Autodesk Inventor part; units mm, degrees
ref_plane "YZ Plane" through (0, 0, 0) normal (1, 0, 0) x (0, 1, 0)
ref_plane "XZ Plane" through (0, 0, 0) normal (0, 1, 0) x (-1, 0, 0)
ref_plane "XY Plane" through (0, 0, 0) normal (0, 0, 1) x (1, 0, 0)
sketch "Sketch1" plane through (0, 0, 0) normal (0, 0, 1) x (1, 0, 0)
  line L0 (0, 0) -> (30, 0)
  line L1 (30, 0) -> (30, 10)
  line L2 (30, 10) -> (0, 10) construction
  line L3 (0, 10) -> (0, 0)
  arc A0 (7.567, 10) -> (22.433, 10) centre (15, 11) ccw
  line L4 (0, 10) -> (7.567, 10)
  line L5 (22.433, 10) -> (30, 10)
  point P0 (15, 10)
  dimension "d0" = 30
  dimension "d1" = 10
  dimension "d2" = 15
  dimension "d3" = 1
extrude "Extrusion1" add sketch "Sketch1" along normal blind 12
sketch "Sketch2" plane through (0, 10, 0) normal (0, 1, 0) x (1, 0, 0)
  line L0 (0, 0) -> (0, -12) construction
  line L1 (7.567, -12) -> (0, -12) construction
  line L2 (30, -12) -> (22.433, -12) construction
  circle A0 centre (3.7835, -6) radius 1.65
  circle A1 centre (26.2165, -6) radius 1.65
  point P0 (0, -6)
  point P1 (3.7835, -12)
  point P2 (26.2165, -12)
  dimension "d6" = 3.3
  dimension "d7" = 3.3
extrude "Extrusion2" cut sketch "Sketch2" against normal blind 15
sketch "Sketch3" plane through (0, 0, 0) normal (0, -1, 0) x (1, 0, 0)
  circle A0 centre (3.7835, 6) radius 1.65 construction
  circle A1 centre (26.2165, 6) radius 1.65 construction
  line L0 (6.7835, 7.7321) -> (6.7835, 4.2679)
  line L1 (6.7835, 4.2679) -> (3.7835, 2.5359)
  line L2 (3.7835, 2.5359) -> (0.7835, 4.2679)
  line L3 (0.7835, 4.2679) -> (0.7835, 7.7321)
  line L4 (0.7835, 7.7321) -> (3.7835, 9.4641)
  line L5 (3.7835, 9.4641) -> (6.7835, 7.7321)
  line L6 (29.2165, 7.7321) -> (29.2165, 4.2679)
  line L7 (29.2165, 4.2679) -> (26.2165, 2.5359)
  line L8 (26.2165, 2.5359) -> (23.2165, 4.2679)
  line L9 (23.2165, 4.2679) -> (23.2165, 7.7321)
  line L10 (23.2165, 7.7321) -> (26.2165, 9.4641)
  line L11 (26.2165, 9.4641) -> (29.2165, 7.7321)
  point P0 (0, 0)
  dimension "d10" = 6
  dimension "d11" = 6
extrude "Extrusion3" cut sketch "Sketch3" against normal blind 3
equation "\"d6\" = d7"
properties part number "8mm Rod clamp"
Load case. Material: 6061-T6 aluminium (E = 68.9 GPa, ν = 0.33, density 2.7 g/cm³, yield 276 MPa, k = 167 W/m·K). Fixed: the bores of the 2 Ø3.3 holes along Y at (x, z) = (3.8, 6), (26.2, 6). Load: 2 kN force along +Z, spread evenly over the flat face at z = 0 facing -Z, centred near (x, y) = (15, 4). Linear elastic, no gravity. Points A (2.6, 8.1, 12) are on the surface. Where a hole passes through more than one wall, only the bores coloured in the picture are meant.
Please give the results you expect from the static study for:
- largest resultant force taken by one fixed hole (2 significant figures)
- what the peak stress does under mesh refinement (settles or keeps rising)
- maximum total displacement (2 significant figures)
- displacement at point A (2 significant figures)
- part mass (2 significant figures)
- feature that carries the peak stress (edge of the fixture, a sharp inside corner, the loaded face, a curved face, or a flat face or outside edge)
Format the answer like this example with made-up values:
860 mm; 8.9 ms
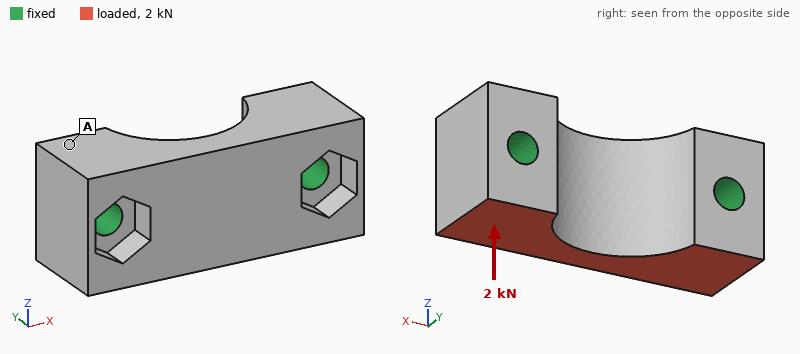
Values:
1.0 kN; keeps rising; 6.6 µm; 1.3 µm; 6.5 g; edge of the fixture
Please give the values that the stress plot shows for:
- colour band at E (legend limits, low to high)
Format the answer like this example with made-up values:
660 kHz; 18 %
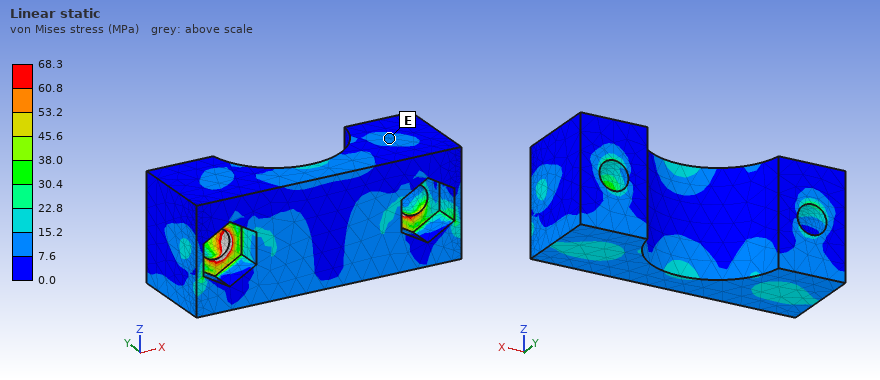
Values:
7.6 to 15.2 MPa
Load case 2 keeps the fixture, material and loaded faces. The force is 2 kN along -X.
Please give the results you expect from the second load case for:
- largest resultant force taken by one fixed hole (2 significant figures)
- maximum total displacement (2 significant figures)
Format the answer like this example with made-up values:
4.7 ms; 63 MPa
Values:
1.1 kN; 6.6 µm
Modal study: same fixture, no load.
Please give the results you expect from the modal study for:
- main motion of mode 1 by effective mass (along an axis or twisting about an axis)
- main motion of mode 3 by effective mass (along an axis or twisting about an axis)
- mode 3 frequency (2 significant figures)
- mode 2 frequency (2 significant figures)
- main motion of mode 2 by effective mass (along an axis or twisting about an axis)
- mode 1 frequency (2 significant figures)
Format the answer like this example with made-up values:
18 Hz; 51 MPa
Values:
along Z; twisting about X; 67 kHz; 56 kHz; along Y; 41 kHz
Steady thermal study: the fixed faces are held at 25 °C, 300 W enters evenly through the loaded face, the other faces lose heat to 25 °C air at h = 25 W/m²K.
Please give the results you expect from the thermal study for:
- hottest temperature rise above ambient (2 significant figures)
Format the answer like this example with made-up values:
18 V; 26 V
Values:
82 K
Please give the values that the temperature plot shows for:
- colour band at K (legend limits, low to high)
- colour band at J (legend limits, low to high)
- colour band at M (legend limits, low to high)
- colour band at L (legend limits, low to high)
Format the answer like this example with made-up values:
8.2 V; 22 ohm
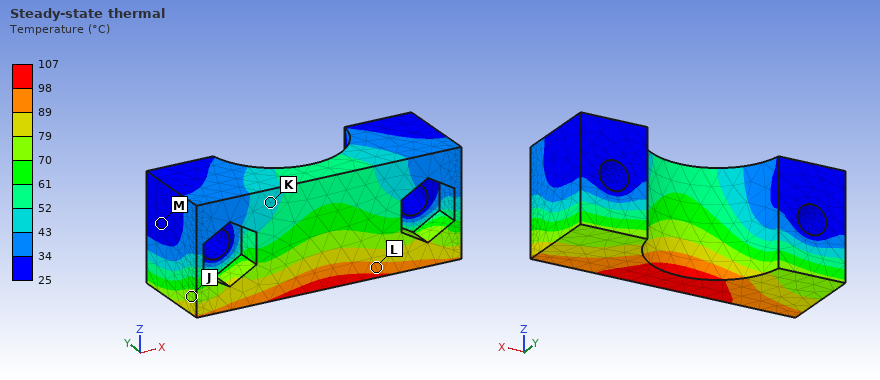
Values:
43 to 52 °C; 70 to 79 °C; 25 to 34 °C; 89 to 98 °C
